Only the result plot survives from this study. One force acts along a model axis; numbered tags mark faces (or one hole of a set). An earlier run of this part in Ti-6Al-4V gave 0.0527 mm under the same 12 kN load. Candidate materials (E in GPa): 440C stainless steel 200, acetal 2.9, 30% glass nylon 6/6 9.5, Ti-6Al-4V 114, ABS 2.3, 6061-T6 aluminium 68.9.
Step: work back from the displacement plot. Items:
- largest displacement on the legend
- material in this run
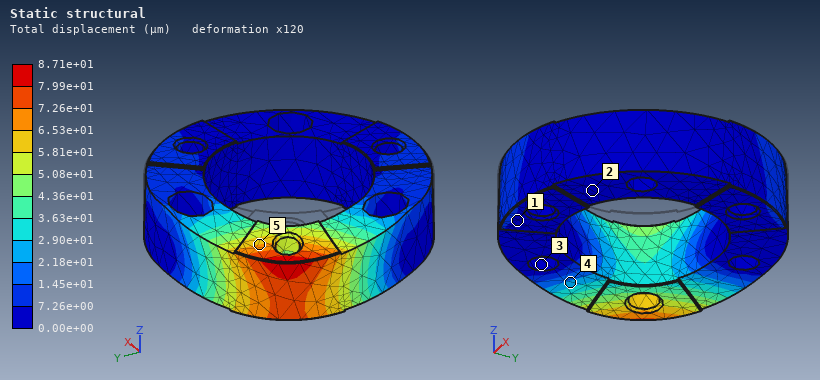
8.71e+01 µm
6061-T6 aluminium
